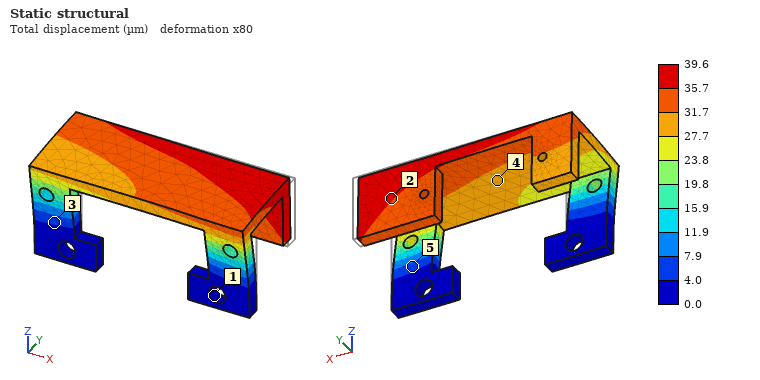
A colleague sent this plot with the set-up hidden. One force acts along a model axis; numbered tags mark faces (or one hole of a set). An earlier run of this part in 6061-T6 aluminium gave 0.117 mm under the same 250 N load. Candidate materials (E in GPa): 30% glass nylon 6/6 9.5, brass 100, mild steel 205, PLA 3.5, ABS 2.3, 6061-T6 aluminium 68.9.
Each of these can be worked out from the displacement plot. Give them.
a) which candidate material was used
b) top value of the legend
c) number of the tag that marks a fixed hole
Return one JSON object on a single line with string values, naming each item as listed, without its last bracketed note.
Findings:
{"which candidate material was used": "mild steel", "top value of the legend": "39.6 µm", "number of the tag that marks a fixed hole": "1"}
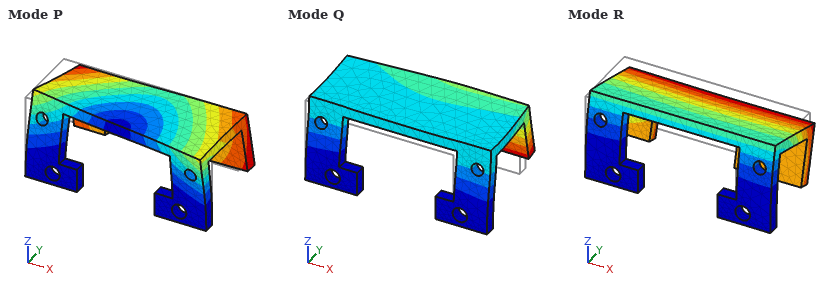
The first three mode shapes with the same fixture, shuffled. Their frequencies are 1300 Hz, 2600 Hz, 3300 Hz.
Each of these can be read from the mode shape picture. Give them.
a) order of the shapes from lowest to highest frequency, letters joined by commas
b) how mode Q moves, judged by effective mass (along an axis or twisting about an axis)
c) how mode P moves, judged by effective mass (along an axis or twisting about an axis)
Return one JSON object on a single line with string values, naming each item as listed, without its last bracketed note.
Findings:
{"order of the shapes from lowest to highest frequency, letters joined by commas": "R, P, Q", "how mode Q moves, judged by effective mass": "along Y", "how mode P moves, judged by effective mass": "along X"}
